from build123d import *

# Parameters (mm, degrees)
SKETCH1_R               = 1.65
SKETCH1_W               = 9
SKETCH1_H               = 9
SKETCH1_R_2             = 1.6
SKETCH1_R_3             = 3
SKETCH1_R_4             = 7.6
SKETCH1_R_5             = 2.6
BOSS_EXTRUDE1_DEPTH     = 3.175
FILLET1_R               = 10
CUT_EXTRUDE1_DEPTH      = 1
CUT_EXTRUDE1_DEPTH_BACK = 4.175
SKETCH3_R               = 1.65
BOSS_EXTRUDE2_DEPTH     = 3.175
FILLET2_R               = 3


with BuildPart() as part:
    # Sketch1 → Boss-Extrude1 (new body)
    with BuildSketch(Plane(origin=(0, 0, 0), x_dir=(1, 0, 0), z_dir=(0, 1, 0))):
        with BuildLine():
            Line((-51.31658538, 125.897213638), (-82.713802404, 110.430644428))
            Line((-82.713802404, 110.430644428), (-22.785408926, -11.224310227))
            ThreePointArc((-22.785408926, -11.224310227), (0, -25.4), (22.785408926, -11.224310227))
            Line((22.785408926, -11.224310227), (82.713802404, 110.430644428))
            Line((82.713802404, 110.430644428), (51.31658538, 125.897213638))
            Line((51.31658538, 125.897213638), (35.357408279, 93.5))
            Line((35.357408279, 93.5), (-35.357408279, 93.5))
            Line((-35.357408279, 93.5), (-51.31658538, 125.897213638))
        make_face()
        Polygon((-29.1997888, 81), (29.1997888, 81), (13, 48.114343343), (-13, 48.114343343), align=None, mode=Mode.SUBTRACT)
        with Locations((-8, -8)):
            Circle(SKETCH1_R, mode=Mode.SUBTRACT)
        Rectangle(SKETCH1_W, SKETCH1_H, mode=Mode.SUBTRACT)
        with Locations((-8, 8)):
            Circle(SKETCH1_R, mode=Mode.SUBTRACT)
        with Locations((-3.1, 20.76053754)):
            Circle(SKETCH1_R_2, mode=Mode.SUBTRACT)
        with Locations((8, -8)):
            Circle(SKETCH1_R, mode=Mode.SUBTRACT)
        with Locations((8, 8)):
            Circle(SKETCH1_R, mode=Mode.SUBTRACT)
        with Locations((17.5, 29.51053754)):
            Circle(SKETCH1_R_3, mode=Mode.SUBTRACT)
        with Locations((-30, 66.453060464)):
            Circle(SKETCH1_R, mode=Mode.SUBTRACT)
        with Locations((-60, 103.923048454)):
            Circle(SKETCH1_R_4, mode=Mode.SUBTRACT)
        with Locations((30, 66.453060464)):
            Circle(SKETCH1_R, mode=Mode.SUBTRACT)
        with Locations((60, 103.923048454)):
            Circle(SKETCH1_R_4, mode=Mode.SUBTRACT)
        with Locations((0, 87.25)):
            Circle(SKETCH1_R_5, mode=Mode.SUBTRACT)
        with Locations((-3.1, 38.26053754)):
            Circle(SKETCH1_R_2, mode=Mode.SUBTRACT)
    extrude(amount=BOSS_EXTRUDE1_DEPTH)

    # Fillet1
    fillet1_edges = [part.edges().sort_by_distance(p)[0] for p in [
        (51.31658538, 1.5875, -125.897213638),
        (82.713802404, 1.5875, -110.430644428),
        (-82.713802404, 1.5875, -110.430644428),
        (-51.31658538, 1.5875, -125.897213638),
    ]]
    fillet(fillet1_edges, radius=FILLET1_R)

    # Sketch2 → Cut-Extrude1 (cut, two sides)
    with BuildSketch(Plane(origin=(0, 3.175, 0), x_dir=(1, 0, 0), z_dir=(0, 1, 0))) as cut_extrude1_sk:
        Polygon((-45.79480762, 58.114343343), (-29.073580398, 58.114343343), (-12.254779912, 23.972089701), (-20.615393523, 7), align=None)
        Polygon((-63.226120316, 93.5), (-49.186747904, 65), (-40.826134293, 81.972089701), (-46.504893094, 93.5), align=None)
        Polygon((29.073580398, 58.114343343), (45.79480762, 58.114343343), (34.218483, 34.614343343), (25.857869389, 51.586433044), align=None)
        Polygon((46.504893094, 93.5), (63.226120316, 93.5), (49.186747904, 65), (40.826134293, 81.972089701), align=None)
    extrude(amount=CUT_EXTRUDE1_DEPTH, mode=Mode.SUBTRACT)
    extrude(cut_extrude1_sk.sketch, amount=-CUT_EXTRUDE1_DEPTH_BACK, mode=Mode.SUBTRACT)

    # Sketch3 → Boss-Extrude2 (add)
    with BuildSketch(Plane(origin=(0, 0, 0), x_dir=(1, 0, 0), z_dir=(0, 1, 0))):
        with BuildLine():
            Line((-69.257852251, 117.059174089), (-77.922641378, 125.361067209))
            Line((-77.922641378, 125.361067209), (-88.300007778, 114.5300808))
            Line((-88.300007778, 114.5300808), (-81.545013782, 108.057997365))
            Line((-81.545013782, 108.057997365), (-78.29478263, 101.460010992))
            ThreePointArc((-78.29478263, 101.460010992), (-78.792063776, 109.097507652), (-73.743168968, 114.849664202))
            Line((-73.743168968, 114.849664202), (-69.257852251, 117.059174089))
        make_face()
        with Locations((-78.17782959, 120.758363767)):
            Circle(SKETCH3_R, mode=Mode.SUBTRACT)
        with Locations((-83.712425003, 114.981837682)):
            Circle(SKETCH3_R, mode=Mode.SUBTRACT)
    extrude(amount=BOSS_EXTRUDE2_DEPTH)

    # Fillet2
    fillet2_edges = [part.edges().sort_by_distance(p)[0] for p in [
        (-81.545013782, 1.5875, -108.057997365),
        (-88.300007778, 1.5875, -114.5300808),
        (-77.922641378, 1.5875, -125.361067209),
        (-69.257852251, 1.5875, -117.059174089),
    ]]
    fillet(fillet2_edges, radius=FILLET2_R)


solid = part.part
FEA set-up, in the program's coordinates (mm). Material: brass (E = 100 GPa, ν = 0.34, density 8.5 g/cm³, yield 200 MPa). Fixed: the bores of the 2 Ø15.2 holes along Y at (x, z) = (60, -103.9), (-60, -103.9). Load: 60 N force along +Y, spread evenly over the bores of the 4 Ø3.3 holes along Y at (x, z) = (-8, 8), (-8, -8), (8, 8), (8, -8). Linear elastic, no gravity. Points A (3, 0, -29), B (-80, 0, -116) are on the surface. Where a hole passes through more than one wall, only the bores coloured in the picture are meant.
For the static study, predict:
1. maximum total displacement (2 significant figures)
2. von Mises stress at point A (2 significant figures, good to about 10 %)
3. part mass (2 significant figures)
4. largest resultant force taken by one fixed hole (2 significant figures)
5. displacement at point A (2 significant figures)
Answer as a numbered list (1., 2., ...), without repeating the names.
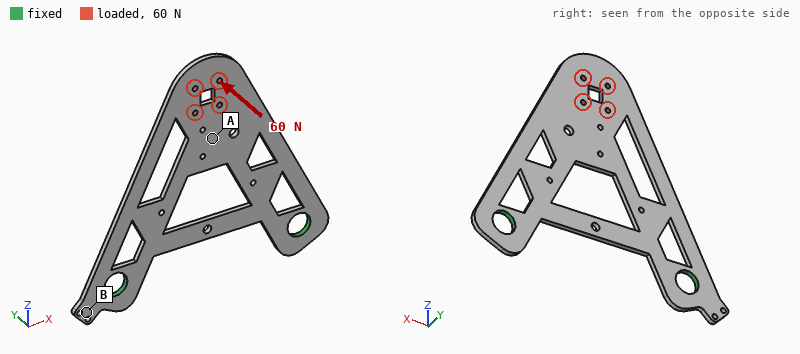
1. 2.4 mm
2. 20 MPa
3. 240 g
4. 31 N
5. 1.1 mm
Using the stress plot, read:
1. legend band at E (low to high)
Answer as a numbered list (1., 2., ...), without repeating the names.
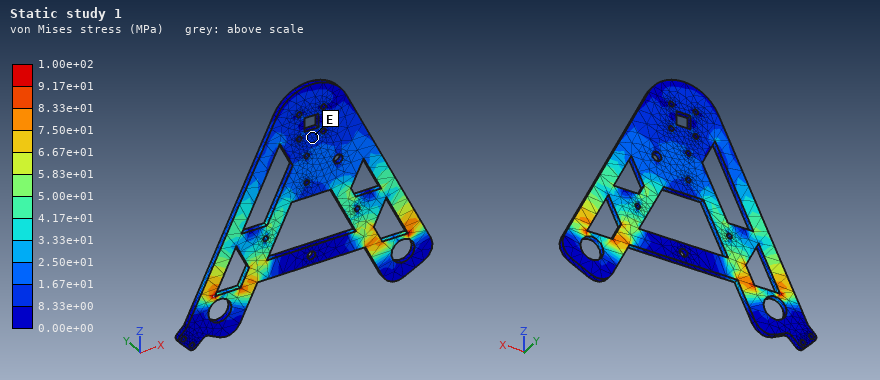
1. 8.33e+00 to 1.67e+01 MPa
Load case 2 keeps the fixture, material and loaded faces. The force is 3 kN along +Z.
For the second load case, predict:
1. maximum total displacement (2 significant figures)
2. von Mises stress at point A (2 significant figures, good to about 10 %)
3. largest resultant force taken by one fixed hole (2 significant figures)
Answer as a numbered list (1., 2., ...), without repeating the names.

1. 34 µm
2. 10.0 MPa
3. 1.7 kN
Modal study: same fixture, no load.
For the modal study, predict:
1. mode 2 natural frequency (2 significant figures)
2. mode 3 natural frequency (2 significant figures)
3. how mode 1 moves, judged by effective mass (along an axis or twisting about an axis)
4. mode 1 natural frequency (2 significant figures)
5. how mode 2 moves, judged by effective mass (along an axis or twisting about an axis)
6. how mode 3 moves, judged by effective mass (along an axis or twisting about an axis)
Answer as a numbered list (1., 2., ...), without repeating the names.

1. 500 Hz
2. 580 Hz
3. along Y
4. 110 Hz
5. twisting about Z
6. along Y
